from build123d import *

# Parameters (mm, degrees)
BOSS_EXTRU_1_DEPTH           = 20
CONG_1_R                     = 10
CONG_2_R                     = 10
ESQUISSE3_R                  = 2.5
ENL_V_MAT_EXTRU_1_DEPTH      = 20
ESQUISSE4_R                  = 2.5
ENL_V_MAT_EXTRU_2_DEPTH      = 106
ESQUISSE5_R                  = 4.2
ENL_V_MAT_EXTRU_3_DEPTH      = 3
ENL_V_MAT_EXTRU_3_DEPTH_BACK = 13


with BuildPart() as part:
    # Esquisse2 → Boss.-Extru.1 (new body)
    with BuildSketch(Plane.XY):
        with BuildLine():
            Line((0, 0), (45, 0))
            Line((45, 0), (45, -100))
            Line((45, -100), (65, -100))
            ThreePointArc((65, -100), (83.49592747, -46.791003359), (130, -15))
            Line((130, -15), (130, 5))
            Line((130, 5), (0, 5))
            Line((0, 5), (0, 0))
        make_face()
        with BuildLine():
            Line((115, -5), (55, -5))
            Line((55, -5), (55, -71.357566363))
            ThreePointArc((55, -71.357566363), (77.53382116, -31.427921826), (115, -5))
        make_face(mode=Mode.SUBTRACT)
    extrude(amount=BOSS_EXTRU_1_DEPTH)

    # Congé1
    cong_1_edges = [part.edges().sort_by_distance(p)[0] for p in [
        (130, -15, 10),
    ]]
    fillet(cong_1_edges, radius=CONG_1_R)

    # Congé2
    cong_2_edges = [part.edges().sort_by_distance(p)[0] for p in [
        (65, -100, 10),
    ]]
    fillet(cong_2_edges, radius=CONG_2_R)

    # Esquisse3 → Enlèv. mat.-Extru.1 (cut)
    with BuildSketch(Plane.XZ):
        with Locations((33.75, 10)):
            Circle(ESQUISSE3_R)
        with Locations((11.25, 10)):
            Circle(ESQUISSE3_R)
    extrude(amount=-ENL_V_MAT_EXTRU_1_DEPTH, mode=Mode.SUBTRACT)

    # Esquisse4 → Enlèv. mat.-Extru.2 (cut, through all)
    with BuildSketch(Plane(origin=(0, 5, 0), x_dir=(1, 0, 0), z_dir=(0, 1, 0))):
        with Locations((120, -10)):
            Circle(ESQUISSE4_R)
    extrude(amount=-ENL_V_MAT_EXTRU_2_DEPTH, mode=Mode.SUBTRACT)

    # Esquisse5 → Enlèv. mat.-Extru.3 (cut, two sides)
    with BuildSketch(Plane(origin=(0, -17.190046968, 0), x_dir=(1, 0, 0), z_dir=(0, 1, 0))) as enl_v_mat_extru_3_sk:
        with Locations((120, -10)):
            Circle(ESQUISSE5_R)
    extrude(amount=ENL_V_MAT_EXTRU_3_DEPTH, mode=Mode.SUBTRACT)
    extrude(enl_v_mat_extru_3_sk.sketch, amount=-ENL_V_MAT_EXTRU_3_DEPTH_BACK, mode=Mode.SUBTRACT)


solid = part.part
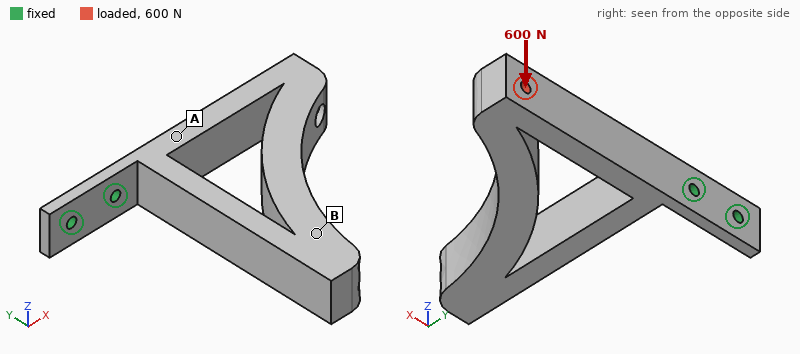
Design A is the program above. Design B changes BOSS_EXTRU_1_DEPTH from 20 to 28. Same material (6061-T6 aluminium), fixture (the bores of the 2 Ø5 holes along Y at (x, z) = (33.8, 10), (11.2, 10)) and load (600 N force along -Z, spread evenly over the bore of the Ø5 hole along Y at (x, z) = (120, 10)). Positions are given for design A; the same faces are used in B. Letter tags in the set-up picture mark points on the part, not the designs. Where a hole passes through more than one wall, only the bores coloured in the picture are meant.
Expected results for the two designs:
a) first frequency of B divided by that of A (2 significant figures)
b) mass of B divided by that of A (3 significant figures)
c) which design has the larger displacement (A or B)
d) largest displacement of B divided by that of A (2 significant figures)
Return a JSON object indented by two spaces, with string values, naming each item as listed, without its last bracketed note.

{
  "first frequency of B divided by that of A": "0.96",
  "mass of B divided by that of A": "1.40",
  "which design has the larger displacement": "A",
  "largest displacement of B divided by that of A": "0.46"
}
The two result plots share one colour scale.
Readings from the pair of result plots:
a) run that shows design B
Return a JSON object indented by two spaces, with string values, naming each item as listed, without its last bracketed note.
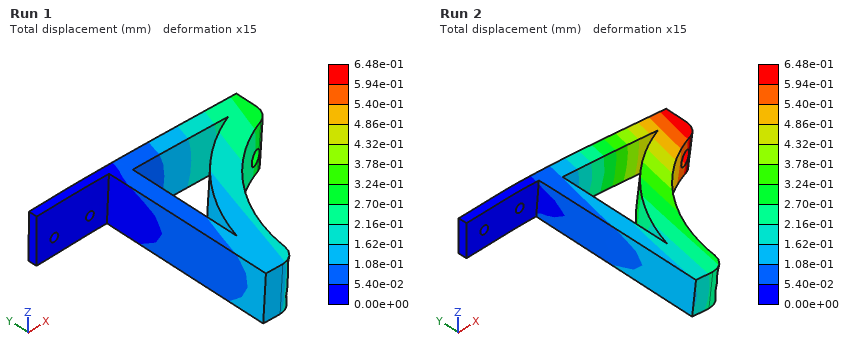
{
  "run that shows design B": "Run 1"
}
